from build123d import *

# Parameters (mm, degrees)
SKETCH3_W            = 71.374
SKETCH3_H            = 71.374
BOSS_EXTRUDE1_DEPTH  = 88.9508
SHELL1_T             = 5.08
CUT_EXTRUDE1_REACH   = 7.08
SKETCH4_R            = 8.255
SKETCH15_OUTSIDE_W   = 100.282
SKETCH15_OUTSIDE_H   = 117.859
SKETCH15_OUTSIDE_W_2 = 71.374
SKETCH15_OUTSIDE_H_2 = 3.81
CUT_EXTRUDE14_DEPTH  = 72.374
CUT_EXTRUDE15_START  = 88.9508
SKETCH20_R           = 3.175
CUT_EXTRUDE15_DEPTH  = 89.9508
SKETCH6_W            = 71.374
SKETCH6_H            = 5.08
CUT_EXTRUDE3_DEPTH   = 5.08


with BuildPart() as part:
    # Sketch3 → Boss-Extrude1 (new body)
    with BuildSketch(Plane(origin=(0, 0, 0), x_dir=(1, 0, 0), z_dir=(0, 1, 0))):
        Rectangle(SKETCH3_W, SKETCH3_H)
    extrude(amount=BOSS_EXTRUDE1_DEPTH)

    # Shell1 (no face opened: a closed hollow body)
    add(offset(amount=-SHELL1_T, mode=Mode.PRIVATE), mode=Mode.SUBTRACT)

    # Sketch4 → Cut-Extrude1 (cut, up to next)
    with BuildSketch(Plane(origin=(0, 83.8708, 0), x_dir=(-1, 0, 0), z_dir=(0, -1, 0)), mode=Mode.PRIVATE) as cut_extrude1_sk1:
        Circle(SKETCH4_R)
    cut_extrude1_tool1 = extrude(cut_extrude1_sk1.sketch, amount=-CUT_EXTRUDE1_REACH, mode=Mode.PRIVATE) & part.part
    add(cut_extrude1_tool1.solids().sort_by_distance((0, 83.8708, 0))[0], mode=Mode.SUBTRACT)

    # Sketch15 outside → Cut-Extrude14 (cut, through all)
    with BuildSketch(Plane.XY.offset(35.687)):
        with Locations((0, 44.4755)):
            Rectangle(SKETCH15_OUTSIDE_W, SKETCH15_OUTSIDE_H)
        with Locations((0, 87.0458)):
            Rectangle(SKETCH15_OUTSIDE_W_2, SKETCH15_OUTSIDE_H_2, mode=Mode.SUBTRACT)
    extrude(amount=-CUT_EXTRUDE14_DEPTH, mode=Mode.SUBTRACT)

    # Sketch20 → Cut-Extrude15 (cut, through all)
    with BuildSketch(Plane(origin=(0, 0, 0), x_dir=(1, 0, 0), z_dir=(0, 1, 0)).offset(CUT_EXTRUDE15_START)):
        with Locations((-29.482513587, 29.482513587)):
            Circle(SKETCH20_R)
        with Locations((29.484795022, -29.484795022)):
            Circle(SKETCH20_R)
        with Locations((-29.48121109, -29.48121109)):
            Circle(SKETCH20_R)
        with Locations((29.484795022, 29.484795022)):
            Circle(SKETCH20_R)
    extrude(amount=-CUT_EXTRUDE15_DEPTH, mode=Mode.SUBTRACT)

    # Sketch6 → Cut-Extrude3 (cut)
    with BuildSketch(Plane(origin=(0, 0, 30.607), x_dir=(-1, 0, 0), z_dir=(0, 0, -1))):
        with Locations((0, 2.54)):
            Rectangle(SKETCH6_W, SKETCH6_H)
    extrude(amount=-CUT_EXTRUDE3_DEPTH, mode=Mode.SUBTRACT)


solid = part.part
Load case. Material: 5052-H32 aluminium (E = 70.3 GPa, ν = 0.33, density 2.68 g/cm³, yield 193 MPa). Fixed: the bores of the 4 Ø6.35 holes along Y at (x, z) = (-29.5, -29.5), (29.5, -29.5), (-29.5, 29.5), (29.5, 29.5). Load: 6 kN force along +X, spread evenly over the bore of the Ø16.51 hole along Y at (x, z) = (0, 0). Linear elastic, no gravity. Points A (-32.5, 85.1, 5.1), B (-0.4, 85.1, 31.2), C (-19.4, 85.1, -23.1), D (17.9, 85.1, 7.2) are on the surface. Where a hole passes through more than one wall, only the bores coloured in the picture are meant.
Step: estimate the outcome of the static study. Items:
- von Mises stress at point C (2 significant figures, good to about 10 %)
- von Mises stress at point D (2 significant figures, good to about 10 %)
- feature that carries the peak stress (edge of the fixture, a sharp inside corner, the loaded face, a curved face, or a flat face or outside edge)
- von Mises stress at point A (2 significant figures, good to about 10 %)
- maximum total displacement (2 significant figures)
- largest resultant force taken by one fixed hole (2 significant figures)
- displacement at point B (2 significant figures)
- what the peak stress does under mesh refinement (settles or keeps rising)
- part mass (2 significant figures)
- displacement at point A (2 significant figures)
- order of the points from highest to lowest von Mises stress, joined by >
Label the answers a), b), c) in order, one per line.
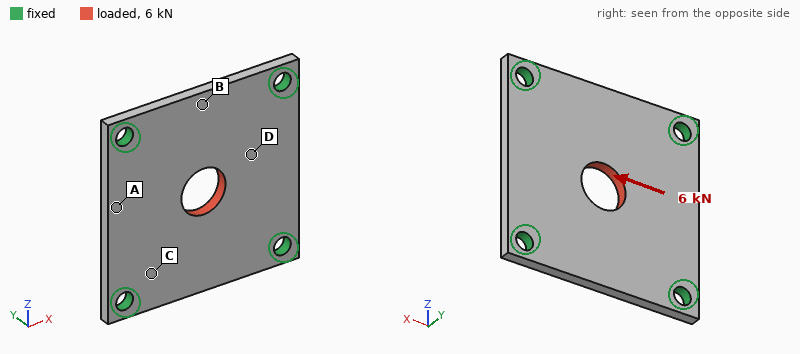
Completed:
a) 26 MPa
b) 19 MPa
c) edge of the fixture
d) 11 MPa
e) 16 µm
f) 1.7 kN
g) 4.1 µm
h) keeps rising
i) 49 g
j) 11 µm
k) C > D > A > B
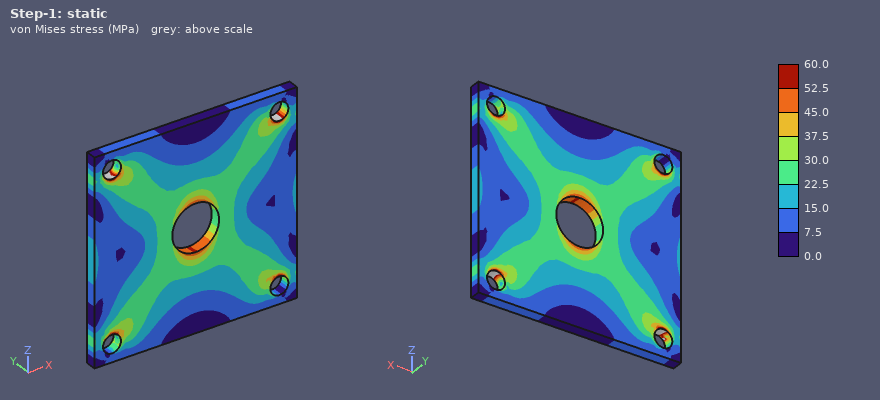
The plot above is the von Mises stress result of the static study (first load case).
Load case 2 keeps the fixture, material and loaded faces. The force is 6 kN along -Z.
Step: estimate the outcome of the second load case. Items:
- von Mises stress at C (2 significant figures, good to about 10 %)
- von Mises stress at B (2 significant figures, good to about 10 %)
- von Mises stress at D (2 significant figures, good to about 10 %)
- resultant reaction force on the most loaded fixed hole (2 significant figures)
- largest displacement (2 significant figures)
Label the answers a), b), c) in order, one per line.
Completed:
a) 26 MPa
b) 10 MPa
c) 20 MPa
d) 1.7 kN
e) 16 µm
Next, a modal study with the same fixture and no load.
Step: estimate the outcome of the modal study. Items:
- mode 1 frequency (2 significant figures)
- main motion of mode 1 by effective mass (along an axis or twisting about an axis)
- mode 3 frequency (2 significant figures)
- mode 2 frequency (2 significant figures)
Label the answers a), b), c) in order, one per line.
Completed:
a) 4200 Hz
b) along Y
c) 6900 Hz
d) 6900 Hz
